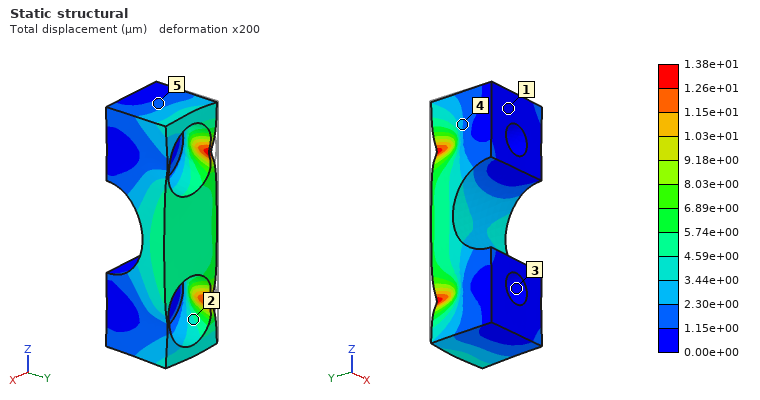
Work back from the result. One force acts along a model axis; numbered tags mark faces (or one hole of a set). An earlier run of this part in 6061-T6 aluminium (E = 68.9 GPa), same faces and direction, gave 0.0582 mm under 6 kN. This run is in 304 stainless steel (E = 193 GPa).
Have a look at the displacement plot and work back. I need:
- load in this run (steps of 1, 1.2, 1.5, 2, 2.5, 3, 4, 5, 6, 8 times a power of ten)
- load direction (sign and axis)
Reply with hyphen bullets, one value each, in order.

- 4 kN
- +X
